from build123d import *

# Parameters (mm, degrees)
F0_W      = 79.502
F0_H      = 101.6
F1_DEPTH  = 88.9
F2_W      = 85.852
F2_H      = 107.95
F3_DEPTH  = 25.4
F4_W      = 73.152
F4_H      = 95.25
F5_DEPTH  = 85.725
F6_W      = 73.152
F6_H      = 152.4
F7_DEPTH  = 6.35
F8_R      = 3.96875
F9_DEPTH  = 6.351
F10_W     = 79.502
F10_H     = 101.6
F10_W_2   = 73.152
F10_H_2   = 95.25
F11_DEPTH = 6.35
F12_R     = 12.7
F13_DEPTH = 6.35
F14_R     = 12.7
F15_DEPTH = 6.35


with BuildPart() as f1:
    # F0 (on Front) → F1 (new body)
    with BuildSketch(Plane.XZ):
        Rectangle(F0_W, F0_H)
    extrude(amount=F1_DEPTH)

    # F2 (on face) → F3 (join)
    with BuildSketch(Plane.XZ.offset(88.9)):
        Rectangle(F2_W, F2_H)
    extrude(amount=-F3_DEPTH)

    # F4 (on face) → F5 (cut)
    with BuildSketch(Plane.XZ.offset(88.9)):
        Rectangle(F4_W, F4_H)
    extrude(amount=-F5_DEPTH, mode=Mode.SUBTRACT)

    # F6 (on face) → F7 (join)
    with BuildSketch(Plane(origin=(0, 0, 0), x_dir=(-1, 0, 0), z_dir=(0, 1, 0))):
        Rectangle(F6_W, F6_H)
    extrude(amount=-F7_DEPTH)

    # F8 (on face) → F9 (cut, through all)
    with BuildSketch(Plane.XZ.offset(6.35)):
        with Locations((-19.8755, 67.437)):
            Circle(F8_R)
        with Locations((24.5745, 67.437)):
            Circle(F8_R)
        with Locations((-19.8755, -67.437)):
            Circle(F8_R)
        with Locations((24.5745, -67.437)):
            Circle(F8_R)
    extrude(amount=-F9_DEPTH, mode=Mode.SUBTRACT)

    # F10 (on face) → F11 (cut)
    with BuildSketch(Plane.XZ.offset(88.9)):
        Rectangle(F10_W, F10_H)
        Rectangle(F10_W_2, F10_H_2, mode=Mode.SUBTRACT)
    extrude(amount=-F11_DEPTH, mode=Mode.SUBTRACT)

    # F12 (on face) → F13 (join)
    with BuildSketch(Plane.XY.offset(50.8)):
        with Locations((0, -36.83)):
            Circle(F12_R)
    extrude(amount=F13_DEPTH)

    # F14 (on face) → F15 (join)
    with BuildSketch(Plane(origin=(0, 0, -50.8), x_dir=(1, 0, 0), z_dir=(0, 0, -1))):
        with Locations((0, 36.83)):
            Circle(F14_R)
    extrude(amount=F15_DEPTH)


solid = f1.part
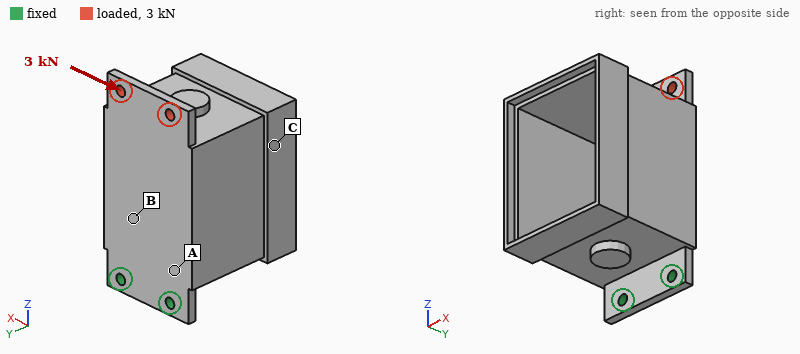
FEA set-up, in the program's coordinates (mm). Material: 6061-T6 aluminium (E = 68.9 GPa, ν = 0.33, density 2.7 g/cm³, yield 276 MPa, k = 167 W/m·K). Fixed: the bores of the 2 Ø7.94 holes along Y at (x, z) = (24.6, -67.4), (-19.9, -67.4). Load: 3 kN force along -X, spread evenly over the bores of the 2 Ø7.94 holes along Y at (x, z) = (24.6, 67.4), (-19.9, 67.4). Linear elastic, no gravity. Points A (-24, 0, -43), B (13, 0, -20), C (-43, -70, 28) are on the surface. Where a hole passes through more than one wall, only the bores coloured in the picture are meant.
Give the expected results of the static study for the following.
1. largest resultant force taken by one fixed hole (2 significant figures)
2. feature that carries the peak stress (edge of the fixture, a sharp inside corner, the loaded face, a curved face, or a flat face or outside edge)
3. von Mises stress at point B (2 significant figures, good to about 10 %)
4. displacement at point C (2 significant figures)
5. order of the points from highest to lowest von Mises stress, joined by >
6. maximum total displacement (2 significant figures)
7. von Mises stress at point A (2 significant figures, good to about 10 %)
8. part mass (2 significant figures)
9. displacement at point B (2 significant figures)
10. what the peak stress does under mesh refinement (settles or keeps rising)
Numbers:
8.4 kN
edge of the fixture
21 MPa
0.13 mm
A > B > C
0.22 mm
36 MPa
530 g
0.054 mm
keeps rising
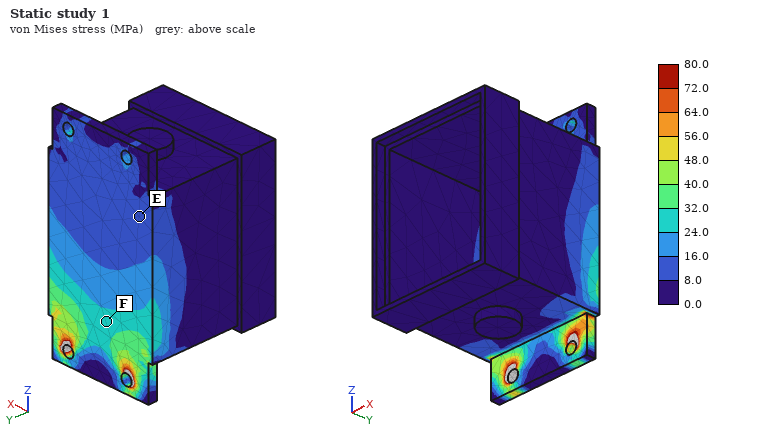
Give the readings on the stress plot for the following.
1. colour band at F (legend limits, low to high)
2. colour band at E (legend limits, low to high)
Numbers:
24.0 to 32.0 MPa
8.0 to 16.0 MPa
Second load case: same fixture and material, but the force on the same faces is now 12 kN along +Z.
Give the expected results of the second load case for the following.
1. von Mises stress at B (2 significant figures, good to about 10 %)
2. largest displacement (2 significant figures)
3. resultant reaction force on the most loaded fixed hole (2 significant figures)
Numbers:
25 MPa
90 µm
6.1 kN
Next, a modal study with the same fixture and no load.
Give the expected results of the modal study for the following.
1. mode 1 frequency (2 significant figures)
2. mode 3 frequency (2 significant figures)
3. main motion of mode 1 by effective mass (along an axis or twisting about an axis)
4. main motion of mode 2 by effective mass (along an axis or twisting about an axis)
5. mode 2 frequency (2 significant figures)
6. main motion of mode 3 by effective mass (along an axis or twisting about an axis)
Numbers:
180 Hz
1600 Hz
along Y
along X
580 Hz
along X
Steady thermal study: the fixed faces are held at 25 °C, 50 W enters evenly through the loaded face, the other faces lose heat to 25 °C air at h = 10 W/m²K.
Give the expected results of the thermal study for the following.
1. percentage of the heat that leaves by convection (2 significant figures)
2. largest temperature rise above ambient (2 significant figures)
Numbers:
37 %
55 K
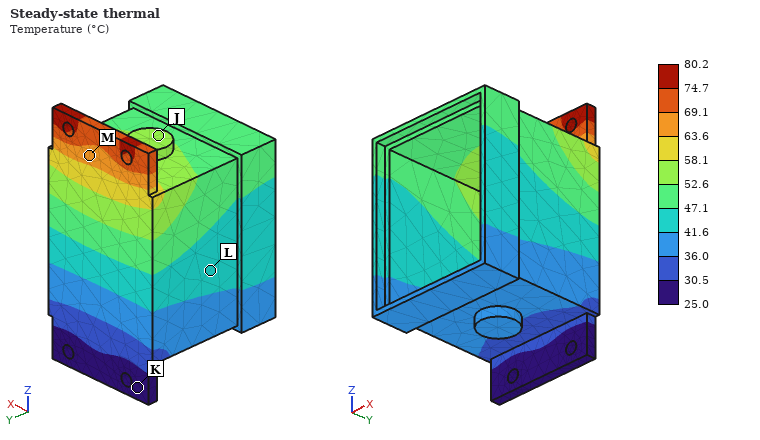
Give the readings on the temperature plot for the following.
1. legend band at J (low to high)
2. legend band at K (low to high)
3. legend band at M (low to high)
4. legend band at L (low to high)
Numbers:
52.6 to 58.1 °C
25.0 to 30.5 °C
63.6 to 69.1 °C
41.6 to 47.1 °C
